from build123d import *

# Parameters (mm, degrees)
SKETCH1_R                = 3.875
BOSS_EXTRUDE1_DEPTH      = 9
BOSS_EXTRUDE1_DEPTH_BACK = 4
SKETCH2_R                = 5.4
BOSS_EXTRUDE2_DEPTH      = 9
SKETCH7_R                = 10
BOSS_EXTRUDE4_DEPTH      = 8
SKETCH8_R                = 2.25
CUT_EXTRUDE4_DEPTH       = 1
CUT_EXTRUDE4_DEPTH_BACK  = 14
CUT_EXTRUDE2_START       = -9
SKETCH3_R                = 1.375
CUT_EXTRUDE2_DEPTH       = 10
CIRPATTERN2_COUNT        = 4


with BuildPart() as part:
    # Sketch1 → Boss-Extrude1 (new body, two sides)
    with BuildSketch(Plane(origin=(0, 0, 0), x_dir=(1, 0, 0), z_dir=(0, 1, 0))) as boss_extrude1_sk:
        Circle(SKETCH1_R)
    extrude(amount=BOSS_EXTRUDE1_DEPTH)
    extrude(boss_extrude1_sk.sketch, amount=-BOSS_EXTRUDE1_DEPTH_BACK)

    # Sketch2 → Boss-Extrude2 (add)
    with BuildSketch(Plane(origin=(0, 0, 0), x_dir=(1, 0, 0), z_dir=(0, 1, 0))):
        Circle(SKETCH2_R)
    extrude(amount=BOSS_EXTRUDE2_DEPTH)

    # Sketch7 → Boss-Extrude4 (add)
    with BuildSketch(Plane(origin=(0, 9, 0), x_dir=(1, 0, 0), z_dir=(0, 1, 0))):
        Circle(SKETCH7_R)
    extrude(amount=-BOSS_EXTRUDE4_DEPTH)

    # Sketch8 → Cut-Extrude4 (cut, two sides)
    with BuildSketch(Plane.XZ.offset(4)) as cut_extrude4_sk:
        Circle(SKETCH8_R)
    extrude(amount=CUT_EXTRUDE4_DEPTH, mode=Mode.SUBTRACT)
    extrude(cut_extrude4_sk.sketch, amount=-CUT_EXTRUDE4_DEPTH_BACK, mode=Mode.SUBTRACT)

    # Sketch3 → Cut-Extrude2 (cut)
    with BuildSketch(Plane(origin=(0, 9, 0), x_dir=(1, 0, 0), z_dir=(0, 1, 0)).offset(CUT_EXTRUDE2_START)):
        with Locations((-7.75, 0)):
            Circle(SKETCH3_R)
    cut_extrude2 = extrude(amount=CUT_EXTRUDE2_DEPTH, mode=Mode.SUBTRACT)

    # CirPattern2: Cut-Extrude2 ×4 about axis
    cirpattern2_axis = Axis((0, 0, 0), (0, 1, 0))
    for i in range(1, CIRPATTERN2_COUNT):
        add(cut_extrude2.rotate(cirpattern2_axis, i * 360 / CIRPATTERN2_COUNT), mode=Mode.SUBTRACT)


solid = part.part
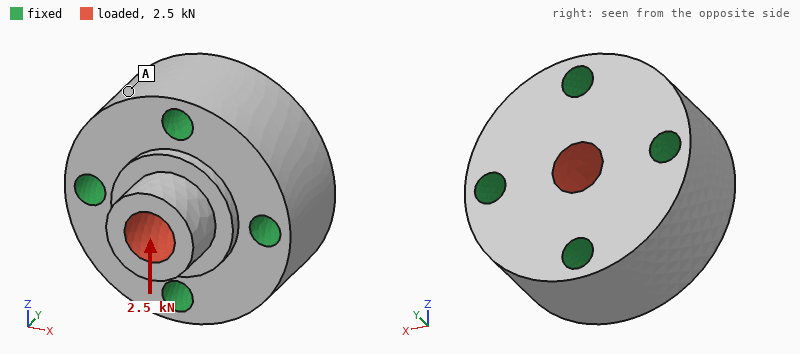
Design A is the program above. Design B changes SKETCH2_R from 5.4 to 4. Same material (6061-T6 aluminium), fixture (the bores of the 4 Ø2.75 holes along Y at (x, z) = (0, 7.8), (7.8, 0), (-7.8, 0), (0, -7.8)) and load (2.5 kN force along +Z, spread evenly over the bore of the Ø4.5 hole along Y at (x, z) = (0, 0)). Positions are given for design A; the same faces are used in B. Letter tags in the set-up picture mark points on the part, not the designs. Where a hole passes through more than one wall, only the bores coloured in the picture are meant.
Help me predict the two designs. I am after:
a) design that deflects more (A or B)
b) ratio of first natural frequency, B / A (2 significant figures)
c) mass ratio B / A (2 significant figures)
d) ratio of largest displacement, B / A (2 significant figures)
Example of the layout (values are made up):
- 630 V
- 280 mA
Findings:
- B
- 0.87
- 0.98
- 1.3
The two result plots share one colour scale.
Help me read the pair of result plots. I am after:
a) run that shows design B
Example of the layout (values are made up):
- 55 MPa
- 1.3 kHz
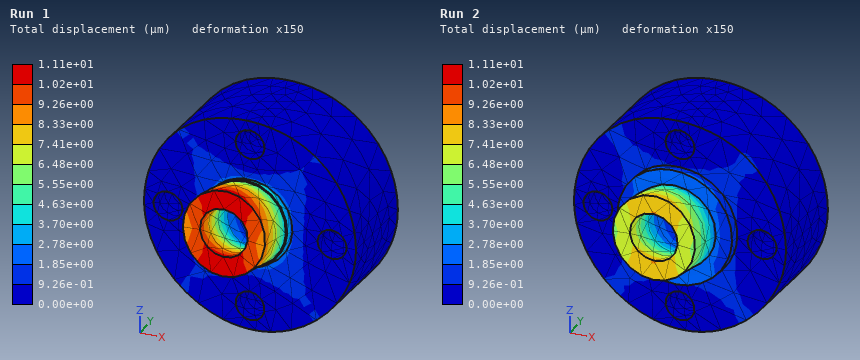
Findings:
- Run 1
